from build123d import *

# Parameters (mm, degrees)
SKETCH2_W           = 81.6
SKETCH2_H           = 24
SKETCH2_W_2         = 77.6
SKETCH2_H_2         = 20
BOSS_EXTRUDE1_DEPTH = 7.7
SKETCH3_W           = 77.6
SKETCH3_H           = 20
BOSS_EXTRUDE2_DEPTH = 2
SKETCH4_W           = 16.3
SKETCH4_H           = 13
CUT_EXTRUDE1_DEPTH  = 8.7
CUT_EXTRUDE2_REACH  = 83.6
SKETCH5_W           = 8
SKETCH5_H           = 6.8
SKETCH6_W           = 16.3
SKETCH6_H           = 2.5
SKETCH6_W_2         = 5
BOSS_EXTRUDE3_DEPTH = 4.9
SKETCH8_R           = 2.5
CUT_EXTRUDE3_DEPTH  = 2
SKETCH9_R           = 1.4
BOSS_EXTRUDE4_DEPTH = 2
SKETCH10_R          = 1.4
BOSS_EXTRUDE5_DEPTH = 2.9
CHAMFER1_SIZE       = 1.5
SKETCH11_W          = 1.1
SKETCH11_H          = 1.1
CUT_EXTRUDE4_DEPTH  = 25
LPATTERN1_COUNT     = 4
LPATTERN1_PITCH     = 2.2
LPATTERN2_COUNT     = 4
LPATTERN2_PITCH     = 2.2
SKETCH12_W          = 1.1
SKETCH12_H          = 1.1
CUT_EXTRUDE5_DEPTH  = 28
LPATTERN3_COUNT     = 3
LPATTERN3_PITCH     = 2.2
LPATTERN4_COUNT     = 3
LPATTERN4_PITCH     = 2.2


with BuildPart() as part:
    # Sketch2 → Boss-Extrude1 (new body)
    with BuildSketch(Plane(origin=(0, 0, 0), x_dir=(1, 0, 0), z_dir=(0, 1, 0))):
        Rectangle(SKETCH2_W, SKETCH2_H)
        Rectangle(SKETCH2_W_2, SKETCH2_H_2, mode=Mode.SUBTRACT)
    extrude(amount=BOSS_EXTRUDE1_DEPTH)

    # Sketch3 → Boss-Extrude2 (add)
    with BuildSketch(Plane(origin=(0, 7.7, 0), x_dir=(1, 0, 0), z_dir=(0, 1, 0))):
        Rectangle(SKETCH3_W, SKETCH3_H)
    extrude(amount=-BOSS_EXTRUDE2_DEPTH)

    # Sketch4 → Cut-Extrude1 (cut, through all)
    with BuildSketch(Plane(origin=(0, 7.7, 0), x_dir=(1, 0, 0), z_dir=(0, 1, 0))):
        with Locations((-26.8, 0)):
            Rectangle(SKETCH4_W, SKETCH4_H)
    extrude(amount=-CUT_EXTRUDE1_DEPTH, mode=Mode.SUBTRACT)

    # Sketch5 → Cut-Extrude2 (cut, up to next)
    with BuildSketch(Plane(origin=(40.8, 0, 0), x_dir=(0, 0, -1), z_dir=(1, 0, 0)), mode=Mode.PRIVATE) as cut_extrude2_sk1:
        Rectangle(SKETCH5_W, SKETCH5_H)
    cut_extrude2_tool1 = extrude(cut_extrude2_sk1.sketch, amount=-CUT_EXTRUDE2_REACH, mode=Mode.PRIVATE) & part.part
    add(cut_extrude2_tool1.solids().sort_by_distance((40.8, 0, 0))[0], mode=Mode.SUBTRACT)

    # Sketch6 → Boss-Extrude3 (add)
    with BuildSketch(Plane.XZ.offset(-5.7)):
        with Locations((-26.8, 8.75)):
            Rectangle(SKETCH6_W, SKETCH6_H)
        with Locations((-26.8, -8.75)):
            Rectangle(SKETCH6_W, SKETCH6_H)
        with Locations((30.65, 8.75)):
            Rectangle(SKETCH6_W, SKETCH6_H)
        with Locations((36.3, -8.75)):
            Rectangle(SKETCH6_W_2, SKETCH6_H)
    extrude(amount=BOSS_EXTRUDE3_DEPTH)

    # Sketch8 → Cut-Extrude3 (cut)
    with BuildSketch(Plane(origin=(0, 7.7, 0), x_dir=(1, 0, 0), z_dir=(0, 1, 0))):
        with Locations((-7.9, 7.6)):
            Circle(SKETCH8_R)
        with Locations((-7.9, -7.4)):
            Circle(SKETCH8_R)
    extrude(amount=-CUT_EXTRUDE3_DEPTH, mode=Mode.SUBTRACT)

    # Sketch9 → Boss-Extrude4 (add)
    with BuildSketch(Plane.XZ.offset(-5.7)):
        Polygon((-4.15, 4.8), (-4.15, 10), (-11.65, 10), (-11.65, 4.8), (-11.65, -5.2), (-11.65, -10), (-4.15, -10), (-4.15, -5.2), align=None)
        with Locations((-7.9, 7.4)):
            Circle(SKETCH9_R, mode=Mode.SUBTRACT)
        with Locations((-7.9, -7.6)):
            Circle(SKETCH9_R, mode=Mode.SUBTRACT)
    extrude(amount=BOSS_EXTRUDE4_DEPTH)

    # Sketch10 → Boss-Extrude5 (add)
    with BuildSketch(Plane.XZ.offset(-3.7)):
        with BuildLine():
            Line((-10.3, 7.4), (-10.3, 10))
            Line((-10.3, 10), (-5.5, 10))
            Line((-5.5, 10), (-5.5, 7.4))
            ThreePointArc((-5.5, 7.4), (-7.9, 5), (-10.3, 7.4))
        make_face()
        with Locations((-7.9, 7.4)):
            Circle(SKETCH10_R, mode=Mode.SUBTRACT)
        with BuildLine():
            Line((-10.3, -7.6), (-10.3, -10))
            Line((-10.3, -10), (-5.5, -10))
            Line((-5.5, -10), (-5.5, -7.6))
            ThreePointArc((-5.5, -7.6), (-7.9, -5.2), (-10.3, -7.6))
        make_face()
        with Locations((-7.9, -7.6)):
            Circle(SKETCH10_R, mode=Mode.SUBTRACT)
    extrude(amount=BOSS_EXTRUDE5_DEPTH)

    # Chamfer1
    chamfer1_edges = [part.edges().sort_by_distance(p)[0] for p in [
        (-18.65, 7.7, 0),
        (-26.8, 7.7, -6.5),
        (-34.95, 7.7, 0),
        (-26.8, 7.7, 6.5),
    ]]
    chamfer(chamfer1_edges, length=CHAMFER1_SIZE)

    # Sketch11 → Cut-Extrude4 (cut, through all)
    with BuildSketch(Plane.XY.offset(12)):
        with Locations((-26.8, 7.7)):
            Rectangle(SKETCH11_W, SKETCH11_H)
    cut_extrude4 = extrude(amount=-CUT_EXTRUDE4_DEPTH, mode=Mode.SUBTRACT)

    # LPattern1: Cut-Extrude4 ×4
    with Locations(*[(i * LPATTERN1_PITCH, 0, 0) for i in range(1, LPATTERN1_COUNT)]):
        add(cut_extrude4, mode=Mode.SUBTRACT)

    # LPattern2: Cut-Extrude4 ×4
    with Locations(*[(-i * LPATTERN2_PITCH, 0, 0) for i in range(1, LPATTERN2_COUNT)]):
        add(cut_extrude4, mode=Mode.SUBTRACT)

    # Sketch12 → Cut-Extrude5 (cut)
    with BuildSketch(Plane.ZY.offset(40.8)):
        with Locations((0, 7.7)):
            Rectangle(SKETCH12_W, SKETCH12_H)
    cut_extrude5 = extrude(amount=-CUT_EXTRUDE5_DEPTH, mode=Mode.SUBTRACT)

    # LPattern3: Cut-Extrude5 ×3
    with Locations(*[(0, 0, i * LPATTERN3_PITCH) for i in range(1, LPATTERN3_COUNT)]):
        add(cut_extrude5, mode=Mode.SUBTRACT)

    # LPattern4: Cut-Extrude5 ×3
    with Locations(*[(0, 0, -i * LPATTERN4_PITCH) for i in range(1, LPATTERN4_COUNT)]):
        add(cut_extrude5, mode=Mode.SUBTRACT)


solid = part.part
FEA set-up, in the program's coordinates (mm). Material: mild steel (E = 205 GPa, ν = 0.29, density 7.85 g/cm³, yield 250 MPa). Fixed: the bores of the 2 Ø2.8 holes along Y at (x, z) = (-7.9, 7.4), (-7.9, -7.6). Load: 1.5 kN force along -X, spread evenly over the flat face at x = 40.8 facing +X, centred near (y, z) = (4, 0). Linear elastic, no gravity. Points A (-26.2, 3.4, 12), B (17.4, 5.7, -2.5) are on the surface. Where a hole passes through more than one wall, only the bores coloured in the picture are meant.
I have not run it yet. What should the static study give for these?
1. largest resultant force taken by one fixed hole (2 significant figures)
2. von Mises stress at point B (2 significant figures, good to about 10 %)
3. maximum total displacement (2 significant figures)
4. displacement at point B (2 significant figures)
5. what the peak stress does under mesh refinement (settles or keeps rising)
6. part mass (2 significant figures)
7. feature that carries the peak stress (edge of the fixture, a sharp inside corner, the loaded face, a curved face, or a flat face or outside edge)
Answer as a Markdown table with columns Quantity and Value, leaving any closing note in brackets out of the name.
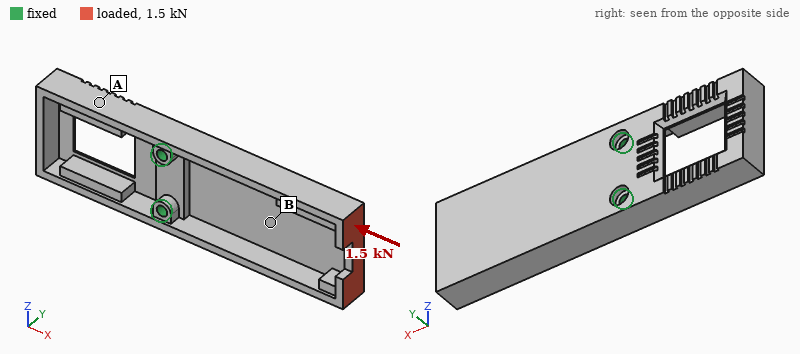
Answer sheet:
| Quantity | Value |
|---|---|
| largest resultant force taken by one fixed hole | 760 N |
| von Mises stress at point B | 20 MPa |
| maximum total displacement | 38 µm |
| displacement at point B | 9.1 µm |
| what the peak stress does under mesh refinement | keeps rising |
| part mass | 52 g |
| feature that carries the peak stress | edge of the fixture |
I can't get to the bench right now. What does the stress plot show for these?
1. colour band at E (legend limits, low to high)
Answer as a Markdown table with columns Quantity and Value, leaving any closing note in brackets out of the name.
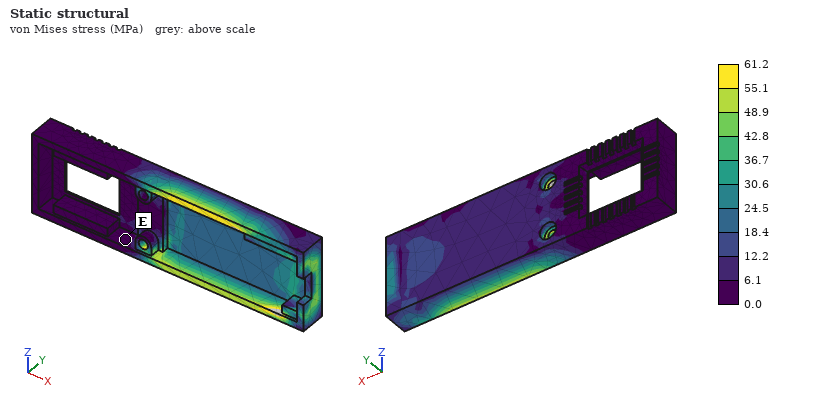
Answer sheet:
| Quantity | Value |
|---|---|
| colour band at E | 0.0 to 6.1 MPa |
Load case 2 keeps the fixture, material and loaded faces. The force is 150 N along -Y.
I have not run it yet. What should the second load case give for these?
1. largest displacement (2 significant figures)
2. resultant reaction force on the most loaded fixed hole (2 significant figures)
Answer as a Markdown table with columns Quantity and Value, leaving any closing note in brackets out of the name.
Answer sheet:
| Quantity | Value |
|---|---|
| largest displacement | 0.13 mm |
| resultant reaction force on the most loaded fixed hole | 83 N |
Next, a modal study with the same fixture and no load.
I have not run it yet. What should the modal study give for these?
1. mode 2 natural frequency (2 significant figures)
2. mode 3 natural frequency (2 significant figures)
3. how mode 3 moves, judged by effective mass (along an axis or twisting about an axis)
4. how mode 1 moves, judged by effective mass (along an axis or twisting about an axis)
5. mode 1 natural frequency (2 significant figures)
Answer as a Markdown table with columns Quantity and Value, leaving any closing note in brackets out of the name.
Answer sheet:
| Quantity | Value |
|---|---|
| mode 2 natural frequency | 3000 Hz |
| mode 3 natural frequency | 3700 Hz |
| how mode 3 moves, judged by effective mass | along Y |
| how mode 1 moves, judged by effective mass | along Y |
| mode 1 natural frequency | 1700 Hz |
